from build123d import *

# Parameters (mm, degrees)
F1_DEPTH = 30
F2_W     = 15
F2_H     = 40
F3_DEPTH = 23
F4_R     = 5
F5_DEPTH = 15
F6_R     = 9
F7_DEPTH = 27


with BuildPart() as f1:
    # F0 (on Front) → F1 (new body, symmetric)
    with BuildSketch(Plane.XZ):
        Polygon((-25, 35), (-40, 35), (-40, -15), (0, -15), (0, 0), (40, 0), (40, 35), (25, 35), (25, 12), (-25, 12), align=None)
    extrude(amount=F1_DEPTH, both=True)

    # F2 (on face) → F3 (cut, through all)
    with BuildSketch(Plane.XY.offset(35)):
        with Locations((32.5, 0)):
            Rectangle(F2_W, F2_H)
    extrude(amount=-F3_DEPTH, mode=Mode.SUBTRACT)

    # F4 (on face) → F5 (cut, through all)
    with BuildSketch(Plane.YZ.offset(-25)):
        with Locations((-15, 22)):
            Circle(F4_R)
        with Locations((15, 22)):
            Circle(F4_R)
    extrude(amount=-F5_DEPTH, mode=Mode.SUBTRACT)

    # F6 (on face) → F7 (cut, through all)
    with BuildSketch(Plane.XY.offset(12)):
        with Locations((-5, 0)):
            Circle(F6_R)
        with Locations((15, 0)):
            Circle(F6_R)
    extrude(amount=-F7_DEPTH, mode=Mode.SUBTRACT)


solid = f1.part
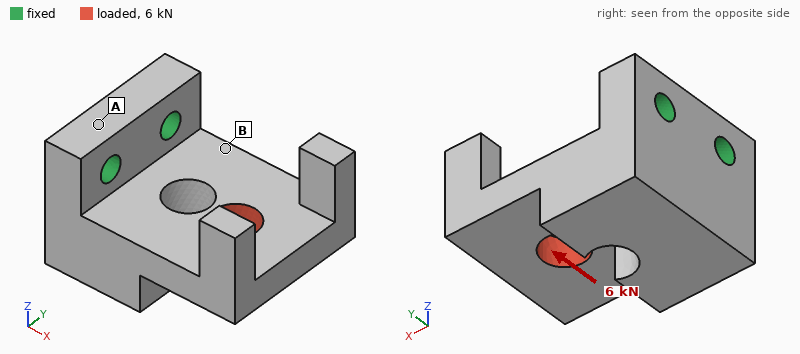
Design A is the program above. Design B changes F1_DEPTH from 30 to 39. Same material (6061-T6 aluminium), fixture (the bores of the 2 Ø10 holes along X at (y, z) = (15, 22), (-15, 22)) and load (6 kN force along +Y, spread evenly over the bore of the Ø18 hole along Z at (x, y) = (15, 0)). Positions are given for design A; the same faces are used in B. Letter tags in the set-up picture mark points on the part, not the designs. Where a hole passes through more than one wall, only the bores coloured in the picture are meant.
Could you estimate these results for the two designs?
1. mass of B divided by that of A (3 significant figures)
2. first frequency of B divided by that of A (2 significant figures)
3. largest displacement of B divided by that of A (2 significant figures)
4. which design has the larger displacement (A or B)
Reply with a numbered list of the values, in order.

1. 1.37
2. 0.91
3. 0.80
4. A
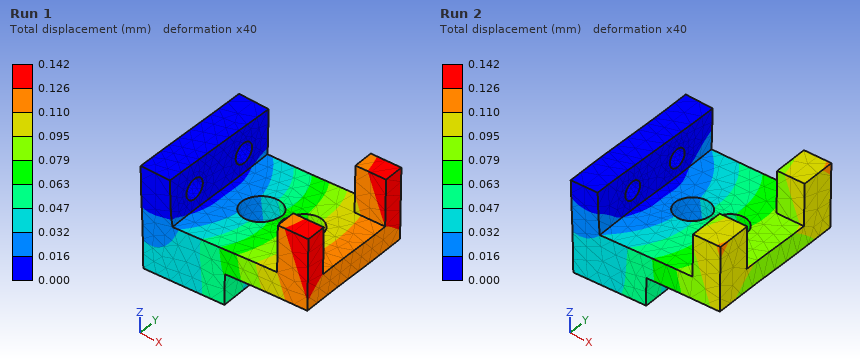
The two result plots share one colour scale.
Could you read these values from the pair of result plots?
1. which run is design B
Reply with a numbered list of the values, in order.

1. Run 2
